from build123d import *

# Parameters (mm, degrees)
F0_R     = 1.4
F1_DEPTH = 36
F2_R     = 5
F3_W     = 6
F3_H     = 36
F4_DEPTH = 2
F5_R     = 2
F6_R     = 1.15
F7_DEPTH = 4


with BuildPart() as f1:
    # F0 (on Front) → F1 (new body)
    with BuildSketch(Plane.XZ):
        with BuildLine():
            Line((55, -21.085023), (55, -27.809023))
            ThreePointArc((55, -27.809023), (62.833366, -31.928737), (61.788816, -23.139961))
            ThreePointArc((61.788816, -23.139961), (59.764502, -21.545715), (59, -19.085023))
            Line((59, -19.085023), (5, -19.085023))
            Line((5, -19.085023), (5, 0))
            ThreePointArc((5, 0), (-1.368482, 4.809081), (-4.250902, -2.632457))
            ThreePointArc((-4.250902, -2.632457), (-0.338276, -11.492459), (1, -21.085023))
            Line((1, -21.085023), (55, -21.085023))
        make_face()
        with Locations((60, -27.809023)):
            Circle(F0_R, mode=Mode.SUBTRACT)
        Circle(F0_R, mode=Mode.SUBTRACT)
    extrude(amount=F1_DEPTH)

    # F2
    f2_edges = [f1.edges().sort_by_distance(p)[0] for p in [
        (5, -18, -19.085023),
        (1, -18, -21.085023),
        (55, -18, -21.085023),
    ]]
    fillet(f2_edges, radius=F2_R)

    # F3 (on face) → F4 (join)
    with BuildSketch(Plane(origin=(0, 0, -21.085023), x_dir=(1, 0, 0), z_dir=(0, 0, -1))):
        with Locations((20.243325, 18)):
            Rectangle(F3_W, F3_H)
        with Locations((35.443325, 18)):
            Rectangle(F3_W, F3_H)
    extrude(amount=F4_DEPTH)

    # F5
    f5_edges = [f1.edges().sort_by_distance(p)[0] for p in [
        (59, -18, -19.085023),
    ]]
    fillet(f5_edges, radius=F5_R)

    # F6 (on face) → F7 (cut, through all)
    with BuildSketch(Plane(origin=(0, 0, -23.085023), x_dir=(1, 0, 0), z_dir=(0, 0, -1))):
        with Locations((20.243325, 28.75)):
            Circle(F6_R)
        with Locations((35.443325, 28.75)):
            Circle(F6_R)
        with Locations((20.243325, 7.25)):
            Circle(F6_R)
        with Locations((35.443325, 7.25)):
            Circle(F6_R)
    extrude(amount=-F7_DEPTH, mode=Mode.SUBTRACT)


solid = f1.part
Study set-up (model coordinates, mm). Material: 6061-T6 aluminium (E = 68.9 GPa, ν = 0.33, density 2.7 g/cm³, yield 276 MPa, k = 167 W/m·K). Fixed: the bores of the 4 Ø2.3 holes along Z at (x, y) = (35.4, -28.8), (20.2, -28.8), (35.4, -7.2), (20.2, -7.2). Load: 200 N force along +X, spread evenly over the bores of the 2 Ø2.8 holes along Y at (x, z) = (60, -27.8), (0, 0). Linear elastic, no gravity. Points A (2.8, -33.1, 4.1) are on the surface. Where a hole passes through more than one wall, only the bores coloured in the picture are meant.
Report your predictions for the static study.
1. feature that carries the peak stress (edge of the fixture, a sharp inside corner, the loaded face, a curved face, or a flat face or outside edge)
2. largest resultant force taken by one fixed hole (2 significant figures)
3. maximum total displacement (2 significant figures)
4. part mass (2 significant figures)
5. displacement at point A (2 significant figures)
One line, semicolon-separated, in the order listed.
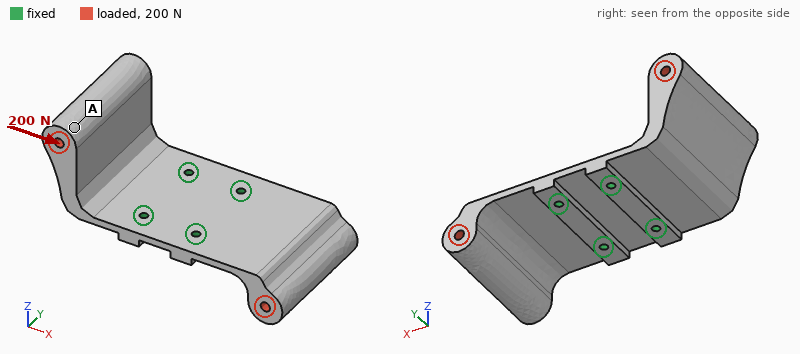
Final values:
a flat face or outside edge; 90 N; 0.37 mm; 38 g; 0.34 mm
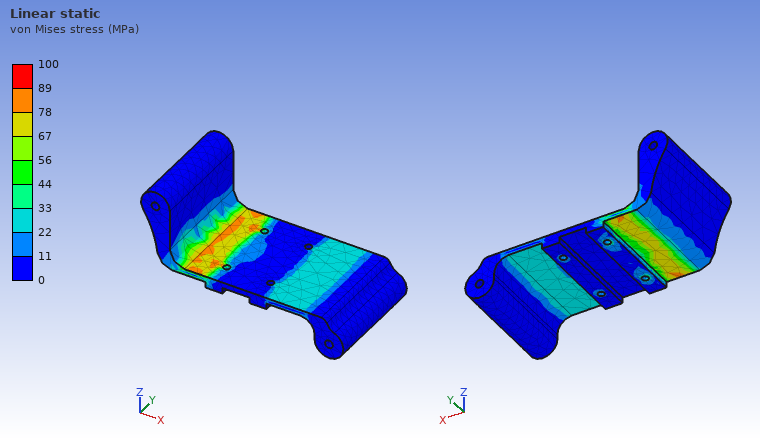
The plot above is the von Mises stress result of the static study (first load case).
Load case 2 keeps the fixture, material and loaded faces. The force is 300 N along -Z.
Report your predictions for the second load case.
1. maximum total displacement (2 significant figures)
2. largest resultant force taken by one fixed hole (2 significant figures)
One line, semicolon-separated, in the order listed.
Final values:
0.46 mm; 130 N
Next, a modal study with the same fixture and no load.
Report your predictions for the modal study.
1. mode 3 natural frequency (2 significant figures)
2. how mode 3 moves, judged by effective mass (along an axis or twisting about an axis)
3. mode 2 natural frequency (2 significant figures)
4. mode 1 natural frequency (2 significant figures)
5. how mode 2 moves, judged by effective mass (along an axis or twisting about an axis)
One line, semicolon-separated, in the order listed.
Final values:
2300 Hz; along Y; 1000 Hz; 810 Hz; along Z
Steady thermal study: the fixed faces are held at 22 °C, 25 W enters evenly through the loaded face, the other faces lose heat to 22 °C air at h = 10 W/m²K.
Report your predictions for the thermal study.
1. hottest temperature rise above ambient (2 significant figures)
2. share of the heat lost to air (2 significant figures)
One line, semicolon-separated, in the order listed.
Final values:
22 K; 4.2 %
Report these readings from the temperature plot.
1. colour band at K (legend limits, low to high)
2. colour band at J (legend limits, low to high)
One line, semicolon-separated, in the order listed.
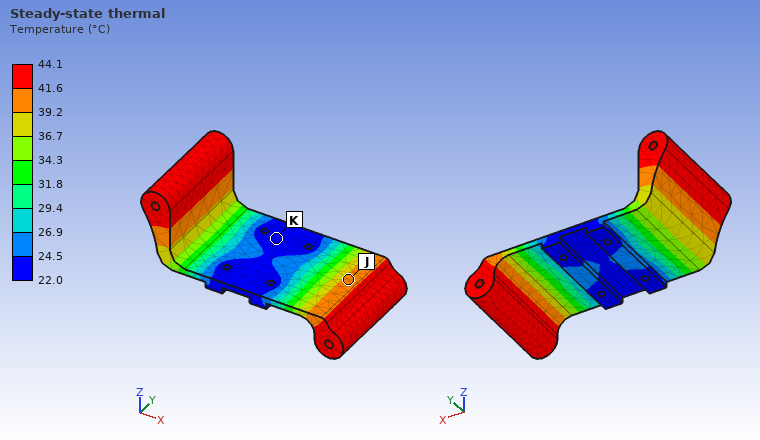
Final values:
22.0 to 24.5 °C; 39.2 to 41.6 °C
